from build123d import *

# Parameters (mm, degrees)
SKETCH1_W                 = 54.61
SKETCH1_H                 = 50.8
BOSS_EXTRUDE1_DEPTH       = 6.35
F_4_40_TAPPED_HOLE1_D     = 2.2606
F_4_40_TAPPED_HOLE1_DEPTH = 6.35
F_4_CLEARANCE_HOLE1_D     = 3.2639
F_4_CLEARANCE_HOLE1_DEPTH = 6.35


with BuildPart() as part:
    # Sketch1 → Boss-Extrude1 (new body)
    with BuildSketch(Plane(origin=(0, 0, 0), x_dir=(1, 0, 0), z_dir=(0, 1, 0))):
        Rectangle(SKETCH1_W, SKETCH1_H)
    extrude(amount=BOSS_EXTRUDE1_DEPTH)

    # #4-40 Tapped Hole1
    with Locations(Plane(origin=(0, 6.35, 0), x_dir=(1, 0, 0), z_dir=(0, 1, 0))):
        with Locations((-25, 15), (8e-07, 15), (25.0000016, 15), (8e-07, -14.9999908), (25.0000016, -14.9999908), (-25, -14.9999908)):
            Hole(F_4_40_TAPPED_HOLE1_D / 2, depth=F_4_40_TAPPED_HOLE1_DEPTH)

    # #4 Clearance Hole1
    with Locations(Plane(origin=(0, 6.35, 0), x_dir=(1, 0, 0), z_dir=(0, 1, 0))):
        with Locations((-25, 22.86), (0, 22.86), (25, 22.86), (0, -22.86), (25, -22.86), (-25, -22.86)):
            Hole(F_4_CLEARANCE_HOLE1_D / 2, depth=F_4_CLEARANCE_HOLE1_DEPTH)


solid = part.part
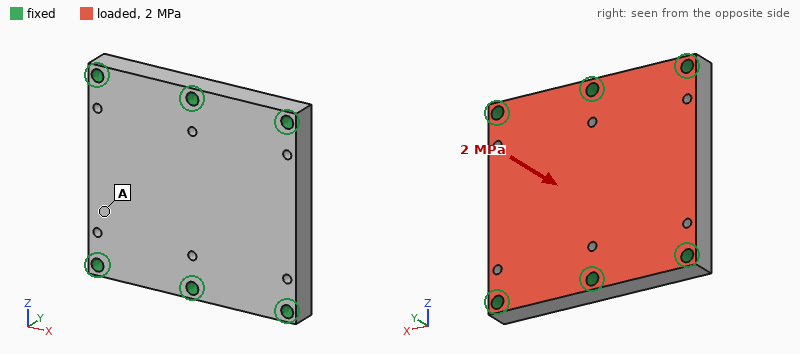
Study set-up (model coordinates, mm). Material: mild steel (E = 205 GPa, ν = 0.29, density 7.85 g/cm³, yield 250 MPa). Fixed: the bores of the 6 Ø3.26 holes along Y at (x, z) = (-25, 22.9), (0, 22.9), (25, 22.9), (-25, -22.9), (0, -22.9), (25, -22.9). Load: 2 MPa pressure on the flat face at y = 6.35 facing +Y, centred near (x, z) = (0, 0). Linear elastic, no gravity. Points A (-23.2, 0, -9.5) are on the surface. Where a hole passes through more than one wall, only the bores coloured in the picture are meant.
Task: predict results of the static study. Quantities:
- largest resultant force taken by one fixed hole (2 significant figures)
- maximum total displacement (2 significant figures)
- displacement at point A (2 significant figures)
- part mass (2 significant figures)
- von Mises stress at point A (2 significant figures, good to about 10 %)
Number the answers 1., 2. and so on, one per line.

1. 1.3 kN
2. 9.0 µm
3. 6.4 µm
4. 130 g
5. 19 MPa
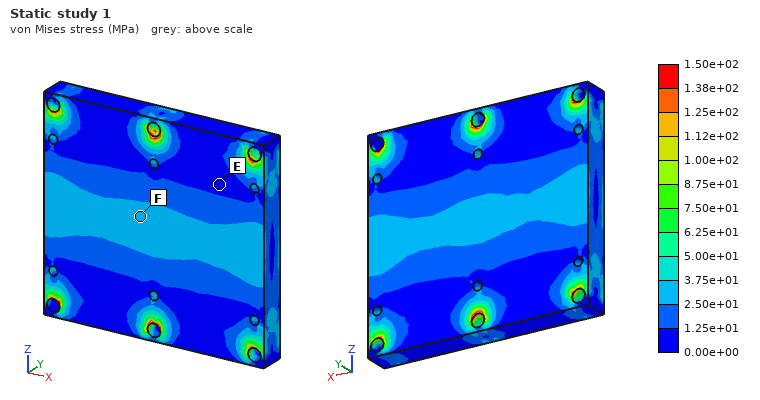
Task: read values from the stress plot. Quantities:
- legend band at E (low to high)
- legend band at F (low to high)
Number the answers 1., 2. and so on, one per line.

1. 0.00e+00 to 1.25e+01 MPa
2. 2.50e+01 to 3.75e+01 MPa
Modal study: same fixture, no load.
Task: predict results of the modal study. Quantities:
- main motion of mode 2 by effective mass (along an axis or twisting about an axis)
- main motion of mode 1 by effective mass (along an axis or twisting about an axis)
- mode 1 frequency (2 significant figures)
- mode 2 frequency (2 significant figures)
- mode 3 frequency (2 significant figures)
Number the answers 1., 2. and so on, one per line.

1. twisting about Z
2. along Y
3. 12 kHz
4. 15 kHz
5. 23 kHz
